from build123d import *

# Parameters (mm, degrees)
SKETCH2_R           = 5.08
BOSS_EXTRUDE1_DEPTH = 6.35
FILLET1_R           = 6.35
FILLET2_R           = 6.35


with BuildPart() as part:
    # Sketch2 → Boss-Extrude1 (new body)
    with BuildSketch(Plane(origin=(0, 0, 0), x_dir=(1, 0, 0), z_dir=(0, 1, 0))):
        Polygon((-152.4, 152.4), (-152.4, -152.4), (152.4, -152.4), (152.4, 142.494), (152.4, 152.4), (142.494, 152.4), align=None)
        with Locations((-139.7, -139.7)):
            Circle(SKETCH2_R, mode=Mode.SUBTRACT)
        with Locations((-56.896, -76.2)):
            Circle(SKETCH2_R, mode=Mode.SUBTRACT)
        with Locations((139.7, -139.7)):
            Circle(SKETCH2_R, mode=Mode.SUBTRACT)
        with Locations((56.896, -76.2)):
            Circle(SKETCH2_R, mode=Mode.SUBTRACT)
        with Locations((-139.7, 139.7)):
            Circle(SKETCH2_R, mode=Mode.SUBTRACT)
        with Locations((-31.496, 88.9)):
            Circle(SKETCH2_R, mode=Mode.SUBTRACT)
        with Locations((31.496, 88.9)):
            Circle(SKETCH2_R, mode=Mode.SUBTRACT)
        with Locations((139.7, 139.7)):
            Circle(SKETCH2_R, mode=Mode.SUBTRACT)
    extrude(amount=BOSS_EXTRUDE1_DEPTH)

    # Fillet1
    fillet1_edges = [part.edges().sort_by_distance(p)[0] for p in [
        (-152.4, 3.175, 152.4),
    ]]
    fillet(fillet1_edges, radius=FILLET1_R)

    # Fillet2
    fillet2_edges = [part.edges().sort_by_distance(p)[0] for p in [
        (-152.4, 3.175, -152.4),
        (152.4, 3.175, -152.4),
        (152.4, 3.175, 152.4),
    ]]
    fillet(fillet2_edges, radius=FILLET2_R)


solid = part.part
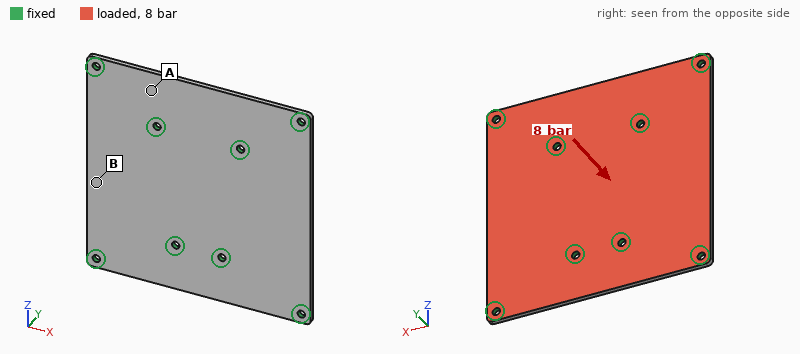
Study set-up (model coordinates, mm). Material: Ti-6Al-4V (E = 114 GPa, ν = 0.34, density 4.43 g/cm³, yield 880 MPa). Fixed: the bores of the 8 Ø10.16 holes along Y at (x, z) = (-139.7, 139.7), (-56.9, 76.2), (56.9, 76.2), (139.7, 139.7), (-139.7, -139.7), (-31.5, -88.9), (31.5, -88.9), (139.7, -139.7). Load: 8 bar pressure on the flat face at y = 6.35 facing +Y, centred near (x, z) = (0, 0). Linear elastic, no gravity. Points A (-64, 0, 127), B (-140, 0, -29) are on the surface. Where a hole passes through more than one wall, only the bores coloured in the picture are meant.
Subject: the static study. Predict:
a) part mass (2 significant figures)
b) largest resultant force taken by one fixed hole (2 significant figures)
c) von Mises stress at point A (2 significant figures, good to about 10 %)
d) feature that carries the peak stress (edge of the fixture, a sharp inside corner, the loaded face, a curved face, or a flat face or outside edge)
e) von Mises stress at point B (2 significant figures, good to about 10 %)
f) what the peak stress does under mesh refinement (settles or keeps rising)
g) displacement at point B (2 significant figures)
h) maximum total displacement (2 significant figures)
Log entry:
2.6 kg
15 kN
82 MPa
edge of the fixture
210 MPa
keeps rising
2.6 mm
3.0 mm
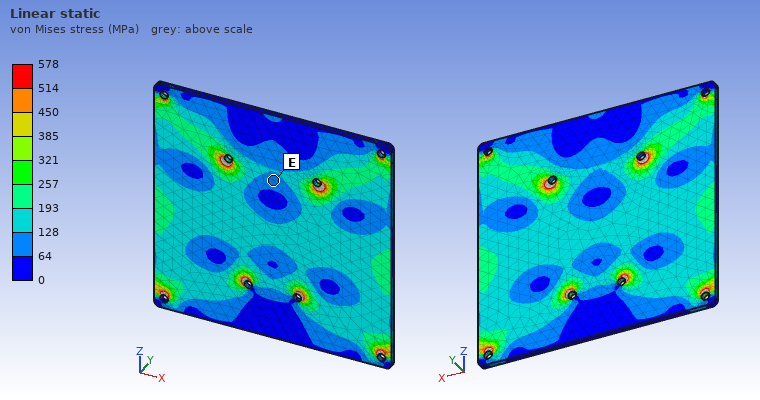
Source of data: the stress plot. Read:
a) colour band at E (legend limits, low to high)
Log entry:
64 to 128 MPa
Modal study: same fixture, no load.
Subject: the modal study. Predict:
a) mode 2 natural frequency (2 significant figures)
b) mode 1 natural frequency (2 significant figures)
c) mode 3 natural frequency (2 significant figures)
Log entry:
640 Hz
640 Hz
1000 Hz
